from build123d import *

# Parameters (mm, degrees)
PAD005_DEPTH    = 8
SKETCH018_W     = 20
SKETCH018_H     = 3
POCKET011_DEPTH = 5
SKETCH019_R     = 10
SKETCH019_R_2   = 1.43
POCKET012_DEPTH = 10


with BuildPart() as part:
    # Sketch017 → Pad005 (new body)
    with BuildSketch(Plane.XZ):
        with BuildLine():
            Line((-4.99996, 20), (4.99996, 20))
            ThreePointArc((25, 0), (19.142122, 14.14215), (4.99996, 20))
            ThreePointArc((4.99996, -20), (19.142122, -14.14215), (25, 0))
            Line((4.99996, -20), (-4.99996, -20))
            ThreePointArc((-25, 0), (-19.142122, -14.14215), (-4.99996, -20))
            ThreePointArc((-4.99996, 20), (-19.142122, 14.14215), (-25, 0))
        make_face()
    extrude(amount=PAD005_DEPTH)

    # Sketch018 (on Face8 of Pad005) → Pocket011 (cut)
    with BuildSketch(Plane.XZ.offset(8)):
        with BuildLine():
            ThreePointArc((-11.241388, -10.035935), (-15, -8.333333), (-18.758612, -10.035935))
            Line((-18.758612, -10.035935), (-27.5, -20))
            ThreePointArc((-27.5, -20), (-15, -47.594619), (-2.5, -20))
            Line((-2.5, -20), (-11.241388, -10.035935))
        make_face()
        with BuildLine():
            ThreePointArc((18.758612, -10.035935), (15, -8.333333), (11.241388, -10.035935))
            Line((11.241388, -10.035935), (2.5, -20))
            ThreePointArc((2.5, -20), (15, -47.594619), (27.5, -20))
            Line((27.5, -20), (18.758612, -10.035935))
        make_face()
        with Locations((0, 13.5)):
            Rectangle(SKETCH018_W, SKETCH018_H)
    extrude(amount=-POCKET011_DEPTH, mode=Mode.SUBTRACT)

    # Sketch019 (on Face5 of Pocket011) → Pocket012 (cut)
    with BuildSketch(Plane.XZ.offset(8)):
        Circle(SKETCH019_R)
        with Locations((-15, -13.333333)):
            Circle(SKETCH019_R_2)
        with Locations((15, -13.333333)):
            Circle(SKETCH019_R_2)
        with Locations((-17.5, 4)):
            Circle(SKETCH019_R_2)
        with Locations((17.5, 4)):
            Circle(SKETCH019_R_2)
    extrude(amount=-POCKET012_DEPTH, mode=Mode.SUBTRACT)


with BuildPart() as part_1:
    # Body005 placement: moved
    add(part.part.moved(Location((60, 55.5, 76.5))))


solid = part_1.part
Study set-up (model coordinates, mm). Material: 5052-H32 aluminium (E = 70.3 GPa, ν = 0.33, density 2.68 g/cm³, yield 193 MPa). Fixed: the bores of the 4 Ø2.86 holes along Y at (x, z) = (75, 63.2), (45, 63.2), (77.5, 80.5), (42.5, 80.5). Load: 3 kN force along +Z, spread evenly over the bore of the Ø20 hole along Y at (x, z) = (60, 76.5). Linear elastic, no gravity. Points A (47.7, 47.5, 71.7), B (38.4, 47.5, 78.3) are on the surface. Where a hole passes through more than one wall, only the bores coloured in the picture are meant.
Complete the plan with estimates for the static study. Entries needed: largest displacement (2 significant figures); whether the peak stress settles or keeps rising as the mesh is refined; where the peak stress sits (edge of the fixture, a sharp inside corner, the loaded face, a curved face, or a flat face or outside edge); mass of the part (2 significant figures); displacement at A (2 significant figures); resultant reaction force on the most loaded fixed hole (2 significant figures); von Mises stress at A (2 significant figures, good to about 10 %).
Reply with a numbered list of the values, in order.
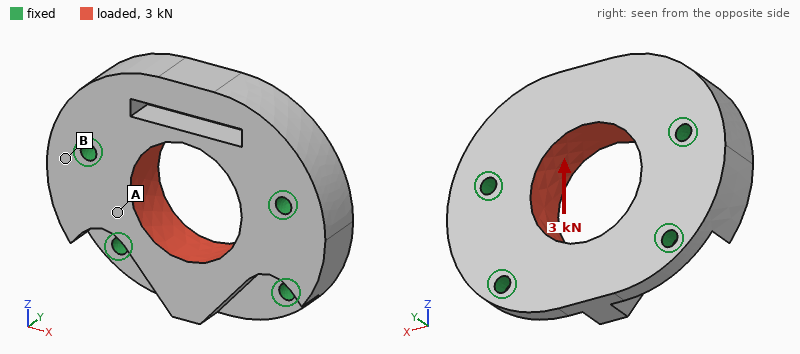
1. 9.8 µm
2. keeps rising
3. edge of the fixture
4. 25 g
5. 2.3 µm
6. 1.1 kN
7. 14 MPa
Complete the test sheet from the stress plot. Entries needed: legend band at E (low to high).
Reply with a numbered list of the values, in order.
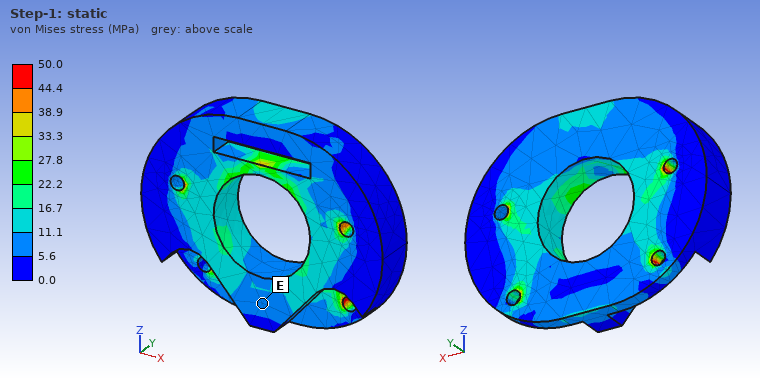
1. 5.6 to 11.1 MPa
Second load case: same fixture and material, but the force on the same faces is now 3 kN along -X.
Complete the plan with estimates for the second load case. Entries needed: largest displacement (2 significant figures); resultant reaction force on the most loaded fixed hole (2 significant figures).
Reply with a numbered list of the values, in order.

1. 3.0 µm
2. 1.1 kN
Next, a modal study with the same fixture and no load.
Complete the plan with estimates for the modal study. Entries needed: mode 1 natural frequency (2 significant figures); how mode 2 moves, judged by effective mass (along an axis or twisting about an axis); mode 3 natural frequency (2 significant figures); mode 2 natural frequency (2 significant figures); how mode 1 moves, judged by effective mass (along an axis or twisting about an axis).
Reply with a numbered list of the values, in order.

1. 16 kHz
2. along Y
3. 30 kHz
4. 20 kHz
5. along Y
